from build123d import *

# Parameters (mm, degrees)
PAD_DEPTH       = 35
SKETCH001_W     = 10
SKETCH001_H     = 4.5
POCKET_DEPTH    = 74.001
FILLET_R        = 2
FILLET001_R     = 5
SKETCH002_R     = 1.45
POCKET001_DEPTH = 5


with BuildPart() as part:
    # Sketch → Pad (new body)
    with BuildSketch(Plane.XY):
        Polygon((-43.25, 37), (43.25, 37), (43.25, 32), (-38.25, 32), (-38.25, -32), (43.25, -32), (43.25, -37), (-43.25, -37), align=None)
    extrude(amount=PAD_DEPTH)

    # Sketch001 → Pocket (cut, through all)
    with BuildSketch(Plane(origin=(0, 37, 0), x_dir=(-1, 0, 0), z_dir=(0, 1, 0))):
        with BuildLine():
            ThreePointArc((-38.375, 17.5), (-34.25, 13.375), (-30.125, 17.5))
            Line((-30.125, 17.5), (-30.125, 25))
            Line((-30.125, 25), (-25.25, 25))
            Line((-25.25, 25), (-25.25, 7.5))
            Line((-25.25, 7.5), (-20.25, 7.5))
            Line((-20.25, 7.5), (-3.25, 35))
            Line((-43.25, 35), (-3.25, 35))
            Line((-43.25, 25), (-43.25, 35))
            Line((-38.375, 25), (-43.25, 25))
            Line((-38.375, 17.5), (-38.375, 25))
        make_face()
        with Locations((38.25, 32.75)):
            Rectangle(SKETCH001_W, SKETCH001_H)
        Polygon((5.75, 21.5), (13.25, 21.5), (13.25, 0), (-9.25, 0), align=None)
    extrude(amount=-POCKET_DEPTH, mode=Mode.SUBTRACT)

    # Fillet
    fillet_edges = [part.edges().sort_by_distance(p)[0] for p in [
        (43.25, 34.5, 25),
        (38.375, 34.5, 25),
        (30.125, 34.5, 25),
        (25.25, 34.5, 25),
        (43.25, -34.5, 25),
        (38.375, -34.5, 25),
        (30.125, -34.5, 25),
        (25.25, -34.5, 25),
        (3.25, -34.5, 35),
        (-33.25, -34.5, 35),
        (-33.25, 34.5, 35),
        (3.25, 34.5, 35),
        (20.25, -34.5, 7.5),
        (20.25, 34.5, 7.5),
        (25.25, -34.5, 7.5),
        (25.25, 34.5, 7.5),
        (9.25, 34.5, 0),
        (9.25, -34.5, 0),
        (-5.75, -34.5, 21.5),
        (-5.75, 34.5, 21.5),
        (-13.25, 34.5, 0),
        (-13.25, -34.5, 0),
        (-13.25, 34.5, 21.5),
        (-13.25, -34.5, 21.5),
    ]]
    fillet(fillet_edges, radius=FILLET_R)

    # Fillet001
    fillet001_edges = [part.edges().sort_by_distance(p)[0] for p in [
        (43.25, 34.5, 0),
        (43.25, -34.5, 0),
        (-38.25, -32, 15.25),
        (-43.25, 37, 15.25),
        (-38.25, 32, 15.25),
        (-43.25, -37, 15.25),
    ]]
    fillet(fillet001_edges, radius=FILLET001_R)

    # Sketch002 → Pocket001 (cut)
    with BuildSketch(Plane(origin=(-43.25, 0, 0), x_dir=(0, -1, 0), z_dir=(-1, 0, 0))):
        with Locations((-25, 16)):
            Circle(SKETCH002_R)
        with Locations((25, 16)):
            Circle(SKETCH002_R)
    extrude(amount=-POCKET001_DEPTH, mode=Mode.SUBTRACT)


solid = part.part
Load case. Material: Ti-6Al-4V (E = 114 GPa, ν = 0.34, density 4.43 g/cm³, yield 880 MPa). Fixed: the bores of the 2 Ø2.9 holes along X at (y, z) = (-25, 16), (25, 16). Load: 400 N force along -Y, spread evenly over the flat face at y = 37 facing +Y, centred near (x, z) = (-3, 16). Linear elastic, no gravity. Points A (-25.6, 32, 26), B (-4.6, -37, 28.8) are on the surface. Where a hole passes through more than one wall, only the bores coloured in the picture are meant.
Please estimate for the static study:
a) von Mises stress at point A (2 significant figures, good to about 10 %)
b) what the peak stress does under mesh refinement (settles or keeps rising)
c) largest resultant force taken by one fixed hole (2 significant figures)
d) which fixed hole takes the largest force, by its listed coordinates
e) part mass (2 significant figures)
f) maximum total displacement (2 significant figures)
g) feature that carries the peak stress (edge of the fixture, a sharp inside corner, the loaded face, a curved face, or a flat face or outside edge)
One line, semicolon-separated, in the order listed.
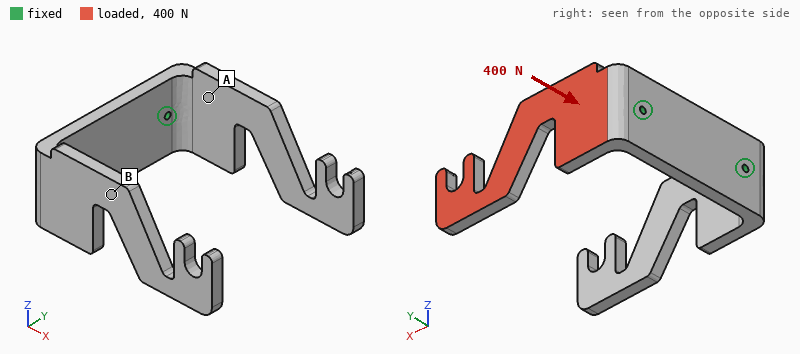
79 MPa; keeps rising; 410 N; (25, 16); 130 g; 1.3 mm; edge of the fixture
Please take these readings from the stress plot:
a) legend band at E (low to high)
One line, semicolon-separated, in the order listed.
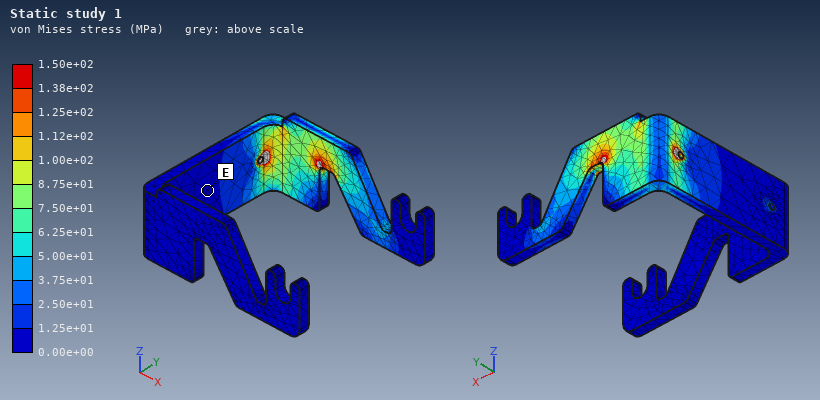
0.00e+00 to 1.25e+01 MPa
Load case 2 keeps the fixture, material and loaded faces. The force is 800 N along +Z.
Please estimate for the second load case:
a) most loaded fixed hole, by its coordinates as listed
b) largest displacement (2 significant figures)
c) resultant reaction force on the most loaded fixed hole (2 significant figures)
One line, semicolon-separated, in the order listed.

(25, 16); 0.68 mm; 970 N
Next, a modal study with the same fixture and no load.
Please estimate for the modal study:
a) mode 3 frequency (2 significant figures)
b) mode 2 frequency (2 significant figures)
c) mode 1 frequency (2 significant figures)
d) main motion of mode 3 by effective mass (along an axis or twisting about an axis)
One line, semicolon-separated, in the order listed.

1000 Hz; 560 Hz; 550 Hz; along Z
